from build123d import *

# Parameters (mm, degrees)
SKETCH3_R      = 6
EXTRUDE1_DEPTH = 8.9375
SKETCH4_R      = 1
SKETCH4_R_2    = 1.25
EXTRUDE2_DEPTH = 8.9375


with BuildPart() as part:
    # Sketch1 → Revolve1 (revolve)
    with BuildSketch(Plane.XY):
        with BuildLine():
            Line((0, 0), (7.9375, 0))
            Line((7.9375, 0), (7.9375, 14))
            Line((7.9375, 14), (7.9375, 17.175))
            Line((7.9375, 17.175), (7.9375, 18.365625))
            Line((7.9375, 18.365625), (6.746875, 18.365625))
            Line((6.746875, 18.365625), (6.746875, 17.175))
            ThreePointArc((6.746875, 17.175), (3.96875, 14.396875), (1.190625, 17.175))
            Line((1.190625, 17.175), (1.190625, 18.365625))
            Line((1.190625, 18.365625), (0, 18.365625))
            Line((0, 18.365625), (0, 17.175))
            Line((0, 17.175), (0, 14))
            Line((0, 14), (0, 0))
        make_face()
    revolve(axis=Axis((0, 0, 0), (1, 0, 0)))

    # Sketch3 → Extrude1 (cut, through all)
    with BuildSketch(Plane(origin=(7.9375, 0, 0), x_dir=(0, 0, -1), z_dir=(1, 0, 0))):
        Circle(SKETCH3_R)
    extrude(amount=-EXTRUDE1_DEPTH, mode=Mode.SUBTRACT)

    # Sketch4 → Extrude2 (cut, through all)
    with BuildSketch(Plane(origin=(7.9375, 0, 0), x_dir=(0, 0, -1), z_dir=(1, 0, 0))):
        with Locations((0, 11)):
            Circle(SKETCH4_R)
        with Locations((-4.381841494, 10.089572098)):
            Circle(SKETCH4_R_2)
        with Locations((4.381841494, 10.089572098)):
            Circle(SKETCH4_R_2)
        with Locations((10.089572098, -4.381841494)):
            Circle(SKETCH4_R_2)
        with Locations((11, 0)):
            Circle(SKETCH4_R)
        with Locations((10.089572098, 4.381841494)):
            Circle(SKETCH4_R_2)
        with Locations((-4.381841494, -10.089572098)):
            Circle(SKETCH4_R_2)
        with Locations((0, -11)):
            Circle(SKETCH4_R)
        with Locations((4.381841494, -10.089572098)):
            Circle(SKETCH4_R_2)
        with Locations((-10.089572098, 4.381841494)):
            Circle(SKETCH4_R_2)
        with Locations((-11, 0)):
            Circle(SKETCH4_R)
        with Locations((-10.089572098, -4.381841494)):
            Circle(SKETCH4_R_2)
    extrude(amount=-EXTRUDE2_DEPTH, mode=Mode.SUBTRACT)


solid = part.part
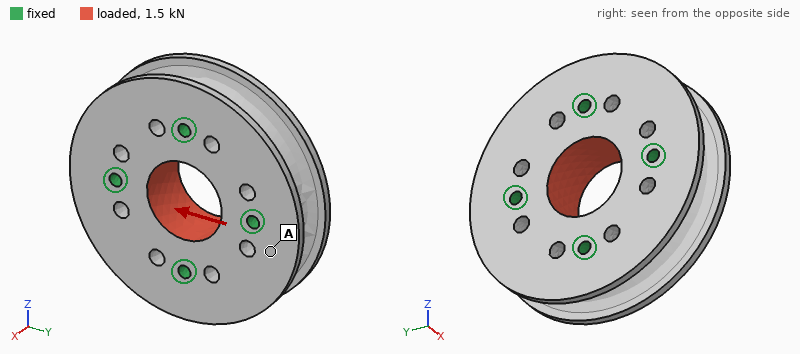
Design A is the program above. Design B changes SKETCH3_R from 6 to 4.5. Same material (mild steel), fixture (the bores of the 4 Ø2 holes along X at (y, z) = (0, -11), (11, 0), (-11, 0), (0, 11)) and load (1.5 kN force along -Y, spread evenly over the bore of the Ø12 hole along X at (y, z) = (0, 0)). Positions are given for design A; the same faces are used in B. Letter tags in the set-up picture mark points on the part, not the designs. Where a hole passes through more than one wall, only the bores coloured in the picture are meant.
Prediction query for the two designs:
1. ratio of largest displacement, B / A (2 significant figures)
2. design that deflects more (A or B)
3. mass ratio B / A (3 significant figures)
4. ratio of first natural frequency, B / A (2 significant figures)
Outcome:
1.1
B
1.08
1.0
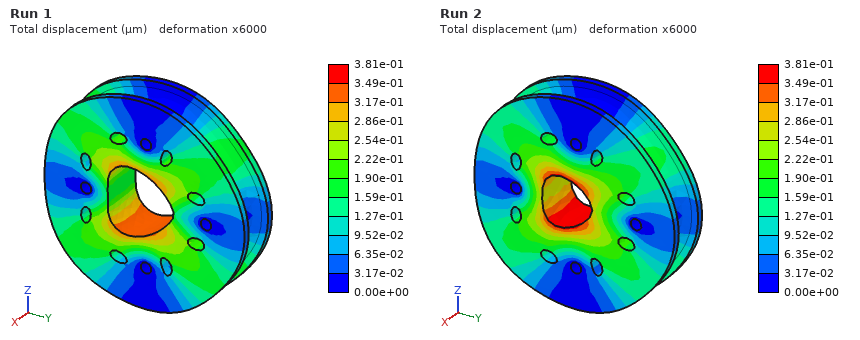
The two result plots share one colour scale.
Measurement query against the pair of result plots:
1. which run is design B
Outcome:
Run 2
